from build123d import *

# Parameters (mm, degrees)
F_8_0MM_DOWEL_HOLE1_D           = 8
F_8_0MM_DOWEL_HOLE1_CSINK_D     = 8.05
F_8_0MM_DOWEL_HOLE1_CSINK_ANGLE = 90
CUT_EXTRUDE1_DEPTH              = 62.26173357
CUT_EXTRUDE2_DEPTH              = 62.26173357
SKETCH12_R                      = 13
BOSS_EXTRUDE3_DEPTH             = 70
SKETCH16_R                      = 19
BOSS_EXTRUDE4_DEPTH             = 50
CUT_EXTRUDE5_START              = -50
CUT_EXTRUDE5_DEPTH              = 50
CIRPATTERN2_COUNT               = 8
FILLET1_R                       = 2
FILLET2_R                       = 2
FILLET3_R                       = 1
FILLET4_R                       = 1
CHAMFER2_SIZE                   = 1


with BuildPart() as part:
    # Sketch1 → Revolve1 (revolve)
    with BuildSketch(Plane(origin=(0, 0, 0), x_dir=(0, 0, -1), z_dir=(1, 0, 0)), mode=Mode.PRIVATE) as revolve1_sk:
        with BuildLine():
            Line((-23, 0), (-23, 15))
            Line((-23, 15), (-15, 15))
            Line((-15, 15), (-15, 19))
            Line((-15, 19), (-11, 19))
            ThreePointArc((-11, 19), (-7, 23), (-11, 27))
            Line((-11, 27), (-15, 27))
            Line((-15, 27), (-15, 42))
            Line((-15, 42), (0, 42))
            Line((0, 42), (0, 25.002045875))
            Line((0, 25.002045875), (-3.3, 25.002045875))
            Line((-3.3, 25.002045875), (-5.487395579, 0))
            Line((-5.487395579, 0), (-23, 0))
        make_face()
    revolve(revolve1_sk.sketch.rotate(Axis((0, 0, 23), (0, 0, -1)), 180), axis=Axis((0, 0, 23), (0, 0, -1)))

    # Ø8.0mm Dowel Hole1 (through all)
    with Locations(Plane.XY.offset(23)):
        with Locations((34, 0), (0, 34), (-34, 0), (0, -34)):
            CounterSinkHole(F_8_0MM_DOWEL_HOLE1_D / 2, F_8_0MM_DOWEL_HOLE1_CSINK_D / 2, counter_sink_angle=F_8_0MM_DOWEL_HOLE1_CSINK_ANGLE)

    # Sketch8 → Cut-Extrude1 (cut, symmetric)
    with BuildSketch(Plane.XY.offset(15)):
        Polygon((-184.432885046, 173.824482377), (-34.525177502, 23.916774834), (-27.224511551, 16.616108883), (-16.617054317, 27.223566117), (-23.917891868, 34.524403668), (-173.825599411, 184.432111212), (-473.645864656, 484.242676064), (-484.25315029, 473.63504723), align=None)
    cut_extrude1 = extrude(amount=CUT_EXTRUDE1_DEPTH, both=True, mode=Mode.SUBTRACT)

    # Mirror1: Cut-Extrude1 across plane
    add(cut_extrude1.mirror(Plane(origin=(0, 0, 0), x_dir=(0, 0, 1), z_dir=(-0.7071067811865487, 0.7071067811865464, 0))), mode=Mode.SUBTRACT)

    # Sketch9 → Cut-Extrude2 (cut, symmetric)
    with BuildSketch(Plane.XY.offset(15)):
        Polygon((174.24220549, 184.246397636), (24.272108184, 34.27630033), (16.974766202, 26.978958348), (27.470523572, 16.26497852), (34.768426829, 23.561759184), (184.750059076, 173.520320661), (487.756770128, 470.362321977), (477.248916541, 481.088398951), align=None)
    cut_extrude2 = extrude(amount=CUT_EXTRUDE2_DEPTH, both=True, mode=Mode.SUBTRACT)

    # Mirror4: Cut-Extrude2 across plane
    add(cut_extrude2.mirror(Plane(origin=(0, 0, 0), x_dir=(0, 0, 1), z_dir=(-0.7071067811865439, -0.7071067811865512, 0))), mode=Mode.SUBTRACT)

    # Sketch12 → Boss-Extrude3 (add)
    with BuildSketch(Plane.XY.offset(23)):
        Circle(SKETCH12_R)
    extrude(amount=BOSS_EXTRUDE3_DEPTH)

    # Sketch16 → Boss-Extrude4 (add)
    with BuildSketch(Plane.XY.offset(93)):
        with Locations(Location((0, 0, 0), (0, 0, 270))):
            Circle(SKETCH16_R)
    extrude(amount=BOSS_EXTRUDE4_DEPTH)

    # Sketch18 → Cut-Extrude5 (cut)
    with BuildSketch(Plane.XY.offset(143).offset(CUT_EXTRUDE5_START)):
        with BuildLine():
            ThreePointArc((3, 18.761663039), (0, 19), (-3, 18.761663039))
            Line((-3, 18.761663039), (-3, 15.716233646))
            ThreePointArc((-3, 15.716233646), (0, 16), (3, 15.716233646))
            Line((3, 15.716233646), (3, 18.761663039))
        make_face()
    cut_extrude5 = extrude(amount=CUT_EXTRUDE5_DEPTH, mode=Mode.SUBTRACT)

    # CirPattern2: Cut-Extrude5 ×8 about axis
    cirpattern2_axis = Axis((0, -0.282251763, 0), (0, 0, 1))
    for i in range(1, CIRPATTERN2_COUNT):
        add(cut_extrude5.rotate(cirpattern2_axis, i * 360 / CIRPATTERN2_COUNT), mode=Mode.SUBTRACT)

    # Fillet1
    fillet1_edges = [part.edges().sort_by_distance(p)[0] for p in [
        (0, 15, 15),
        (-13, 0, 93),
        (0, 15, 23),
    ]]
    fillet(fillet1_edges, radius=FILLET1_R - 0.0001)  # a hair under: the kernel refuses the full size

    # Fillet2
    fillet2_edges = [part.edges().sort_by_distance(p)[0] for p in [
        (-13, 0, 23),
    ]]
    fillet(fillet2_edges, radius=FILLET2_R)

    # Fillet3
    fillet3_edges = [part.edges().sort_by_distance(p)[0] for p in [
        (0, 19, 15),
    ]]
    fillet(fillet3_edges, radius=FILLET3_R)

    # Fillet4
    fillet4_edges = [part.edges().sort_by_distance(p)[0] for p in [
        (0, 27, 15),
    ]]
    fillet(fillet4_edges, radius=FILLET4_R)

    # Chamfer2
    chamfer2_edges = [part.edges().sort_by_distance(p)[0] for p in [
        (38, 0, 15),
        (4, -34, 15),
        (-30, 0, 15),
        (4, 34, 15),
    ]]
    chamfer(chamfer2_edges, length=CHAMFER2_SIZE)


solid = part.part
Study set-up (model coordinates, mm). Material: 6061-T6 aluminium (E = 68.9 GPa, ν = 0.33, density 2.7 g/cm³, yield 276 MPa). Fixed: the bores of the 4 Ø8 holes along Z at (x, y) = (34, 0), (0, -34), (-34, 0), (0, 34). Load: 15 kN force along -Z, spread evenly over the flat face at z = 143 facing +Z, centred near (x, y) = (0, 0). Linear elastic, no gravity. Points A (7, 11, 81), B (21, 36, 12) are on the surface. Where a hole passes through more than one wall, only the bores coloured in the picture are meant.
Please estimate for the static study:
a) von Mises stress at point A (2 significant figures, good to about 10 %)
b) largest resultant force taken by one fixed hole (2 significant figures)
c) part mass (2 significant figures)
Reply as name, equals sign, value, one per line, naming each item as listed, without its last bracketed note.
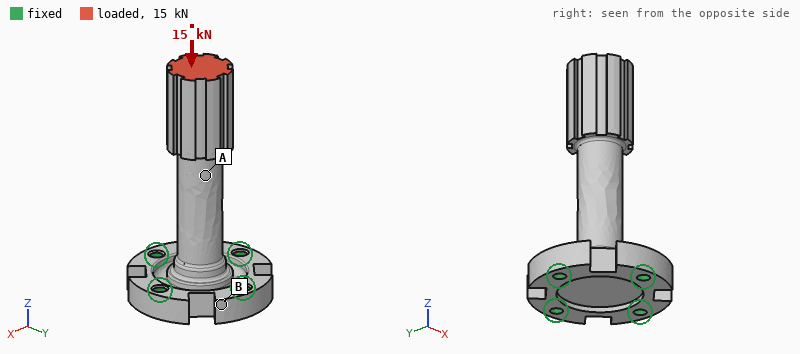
von Mises stress at point A = 27 MPa
largest resultant force taken by one fixed hole = 4.2 kN
part mass = 400 g
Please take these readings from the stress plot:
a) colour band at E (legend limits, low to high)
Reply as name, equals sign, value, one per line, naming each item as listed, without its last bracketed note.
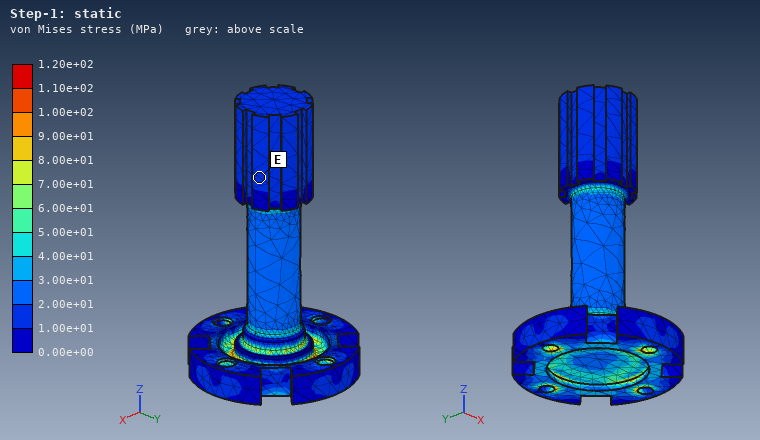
colour band at E = 1.00e+01 to 2.00e+01 MPa
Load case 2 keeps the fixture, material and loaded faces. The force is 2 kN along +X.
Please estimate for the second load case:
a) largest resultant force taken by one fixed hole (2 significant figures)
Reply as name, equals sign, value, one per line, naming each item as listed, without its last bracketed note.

largest resultant force taken by one fixed hole = 5.3 kN
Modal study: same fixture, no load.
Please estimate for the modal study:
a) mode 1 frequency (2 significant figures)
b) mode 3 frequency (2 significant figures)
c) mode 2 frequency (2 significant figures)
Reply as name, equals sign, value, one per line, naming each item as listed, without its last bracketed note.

mode 1 frequency = 680 Hz
mode 3 frequency = 3700 Hz
mode 2 frequency = 680 Hz
